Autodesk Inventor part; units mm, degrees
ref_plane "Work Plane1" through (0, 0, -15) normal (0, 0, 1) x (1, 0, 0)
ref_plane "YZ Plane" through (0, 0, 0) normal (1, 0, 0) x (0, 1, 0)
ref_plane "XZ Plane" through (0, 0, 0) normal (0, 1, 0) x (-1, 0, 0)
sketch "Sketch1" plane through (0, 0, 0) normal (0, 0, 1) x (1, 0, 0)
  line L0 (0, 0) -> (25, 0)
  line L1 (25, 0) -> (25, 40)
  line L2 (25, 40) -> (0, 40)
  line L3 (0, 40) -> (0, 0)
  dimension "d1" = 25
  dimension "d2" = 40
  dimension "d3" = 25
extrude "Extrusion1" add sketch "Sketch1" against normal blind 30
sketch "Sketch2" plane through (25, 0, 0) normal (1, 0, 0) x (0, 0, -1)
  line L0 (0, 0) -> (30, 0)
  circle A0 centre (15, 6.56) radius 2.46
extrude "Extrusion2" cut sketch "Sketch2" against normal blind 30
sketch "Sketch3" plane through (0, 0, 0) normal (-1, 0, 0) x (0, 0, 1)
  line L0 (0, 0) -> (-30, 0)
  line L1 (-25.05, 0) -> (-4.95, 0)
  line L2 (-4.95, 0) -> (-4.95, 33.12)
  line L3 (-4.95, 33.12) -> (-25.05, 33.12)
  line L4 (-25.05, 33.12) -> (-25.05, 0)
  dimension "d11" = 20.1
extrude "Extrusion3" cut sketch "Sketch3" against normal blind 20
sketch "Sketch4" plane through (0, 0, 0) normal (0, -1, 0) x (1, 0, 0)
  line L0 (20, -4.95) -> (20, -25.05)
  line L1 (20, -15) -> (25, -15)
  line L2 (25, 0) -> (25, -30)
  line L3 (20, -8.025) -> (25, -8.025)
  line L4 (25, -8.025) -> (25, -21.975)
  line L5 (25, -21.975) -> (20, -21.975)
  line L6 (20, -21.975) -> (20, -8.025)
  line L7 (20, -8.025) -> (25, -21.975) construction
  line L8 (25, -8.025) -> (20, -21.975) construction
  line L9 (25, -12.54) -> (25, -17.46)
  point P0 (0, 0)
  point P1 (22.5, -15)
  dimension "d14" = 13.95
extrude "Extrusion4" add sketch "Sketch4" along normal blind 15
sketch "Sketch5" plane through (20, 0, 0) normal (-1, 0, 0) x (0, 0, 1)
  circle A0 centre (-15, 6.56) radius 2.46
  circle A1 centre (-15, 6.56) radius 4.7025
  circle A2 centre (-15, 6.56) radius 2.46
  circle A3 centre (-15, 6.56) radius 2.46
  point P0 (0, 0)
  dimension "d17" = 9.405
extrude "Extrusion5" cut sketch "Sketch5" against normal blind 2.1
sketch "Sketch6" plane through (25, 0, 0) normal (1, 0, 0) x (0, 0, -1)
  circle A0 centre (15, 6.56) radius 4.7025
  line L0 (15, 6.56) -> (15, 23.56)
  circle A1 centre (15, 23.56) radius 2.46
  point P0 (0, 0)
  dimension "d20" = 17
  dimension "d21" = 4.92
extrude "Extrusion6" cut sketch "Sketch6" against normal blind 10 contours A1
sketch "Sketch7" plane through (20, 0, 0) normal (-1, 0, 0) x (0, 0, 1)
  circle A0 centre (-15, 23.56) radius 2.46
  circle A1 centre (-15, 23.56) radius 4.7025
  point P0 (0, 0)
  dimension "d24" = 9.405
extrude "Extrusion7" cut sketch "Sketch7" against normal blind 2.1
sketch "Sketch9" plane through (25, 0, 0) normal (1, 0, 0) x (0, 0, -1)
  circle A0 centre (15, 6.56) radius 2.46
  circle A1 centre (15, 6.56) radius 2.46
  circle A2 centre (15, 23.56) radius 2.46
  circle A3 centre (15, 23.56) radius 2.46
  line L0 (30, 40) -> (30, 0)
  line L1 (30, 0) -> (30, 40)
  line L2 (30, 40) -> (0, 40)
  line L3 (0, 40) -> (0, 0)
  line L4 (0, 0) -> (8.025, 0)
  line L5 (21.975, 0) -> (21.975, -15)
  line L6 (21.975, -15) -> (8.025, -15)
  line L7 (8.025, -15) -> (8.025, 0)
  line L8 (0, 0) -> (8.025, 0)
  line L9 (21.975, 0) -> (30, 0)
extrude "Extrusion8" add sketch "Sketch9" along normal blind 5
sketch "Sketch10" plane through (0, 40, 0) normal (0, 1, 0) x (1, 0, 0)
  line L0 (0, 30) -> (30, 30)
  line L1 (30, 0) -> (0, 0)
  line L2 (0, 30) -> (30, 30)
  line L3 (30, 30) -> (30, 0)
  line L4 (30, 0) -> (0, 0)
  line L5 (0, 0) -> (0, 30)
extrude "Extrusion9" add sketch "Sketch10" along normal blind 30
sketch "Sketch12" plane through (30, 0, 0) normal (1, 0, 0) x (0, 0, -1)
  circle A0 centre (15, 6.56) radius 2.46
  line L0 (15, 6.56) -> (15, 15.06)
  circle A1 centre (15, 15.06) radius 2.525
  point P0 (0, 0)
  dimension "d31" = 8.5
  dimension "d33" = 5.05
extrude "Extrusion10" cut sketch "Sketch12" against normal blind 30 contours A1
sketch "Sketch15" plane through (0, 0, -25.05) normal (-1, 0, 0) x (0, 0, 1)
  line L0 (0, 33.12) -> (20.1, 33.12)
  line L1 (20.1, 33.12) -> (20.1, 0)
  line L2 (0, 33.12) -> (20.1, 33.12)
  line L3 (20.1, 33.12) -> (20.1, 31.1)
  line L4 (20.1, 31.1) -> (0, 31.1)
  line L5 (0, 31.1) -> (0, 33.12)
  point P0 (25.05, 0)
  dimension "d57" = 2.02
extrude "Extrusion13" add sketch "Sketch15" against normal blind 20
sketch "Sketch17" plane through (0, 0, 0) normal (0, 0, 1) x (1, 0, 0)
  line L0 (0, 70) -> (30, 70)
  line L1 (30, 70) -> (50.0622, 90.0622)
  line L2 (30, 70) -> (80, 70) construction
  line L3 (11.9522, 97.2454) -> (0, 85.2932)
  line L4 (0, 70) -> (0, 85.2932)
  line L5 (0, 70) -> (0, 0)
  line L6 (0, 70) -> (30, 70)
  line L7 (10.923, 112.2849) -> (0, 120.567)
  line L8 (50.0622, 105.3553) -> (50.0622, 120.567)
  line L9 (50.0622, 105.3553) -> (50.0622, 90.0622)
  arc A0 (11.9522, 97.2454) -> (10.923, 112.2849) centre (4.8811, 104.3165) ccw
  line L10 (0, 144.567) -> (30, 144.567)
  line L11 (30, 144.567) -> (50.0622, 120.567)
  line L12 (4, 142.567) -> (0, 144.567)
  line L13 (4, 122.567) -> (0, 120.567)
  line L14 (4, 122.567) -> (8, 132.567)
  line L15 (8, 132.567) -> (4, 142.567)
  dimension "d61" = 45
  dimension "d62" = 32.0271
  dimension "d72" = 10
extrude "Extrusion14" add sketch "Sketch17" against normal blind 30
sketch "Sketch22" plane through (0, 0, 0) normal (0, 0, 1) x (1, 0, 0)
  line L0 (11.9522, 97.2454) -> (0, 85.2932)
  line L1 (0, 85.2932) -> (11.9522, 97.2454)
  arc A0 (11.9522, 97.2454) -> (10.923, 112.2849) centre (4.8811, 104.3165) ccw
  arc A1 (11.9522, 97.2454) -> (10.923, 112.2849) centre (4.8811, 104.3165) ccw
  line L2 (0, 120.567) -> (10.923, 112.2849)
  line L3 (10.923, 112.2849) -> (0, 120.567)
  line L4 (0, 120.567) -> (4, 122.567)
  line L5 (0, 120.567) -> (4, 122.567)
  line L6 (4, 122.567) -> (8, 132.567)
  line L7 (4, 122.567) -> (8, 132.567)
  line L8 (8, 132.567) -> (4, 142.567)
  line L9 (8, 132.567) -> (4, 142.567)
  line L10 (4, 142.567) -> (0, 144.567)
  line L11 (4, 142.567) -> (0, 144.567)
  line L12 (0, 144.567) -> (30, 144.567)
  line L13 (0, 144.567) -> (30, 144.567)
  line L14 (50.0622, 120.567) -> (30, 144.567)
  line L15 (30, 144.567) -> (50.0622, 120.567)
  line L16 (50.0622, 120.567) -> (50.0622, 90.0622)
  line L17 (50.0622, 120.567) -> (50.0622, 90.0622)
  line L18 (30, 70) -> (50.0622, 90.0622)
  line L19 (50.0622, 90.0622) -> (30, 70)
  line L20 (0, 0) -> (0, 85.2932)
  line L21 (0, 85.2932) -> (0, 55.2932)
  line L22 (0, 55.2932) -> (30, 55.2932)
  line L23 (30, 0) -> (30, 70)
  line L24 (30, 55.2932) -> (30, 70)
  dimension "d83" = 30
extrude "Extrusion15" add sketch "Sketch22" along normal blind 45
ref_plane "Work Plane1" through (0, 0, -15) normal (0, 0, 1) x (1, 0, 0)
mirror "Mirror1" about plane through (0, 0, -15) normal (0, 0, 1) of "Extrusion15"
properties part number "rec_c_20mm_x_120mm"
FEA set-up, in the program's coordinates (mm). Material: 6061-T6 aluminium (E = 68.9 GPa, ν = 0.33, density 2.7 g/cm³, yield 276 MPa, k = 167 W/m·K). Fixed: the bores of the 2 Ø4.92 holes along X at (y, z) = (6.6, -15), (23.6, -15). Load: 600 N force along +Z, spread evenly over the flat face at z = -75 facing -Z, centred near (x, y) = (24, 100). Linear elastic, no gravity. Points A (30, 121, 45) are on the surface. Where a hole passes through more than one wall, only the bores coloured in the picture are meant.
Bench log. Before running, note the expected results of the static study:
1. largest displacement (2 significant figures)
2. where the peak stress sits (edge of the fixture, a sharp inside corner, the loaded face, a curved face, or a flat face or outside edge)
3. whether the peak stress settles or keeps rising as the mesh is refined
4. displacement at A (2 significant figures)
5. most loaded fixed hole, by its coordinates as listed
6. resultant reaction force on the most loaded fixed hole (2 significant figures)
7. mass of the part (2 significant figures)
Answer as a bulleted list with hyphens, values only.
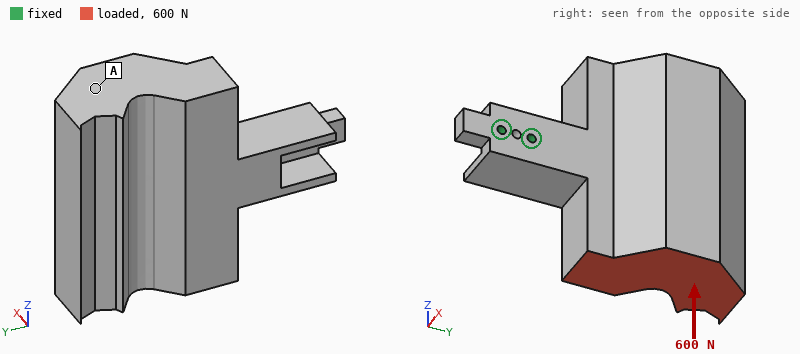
- 0.13 mm
- edge of the fixture
- keeps rising
- 0.11 mm
- (23.6, -15)
- 2.6 kN
- 1.2 kg
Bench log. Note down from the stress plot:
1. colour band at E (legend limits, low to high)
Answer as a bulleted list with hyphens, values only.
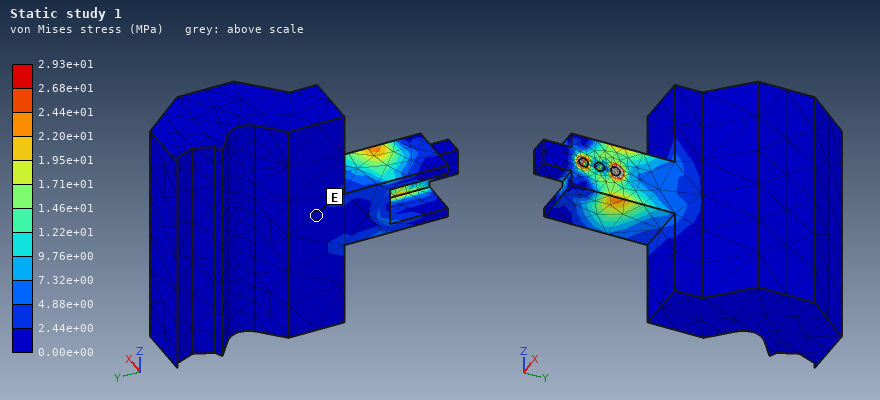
- 0.00e+00 to 2.44e+00 MPa
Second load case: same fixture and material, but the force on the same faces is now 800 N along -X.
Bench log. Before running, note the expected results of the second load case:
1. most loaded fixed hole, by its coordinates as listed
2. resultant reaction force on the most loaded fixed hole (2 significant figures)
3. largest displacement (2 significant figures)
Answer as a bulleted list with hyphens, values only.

- (23.6, -15)
- 3.2 kN
- 0.37 mm
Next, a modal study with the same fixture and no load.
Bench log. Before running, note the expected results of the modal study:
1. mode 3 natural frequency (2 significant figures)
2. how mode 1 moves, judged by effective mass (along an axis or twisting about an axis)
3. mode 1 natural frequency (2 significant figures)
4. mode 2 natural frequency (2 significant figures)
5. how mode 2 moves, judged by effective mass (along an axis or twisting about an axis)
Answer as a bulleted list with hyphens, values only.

- 560 Hz
- along X
- 360 Hz
- 380 Hz
- along Z
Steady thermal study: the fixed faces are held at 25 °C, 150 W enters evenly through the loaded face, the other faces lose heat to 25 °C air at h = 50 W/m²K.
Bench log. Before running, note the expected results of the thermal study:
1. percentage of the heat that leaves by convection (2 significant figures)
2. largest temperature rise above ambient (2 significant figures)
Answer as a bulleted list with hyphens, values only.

- 51 %
- 53 K
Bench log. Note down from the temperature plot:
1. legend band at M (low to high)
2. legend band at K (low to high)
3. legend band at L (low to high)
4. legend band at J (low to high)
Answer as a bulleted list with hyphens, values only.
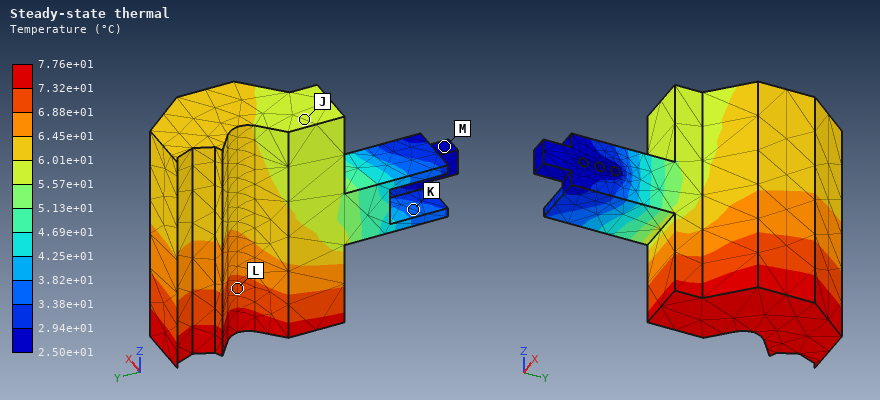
- 2.50e+01 to 2.94e+01 °C
- 3.38e+01 to 3.82e+01 °C
- 6.88e+01 to 7.32e+01 °C
- 5.57e+01 to 6.01e+01 °C
